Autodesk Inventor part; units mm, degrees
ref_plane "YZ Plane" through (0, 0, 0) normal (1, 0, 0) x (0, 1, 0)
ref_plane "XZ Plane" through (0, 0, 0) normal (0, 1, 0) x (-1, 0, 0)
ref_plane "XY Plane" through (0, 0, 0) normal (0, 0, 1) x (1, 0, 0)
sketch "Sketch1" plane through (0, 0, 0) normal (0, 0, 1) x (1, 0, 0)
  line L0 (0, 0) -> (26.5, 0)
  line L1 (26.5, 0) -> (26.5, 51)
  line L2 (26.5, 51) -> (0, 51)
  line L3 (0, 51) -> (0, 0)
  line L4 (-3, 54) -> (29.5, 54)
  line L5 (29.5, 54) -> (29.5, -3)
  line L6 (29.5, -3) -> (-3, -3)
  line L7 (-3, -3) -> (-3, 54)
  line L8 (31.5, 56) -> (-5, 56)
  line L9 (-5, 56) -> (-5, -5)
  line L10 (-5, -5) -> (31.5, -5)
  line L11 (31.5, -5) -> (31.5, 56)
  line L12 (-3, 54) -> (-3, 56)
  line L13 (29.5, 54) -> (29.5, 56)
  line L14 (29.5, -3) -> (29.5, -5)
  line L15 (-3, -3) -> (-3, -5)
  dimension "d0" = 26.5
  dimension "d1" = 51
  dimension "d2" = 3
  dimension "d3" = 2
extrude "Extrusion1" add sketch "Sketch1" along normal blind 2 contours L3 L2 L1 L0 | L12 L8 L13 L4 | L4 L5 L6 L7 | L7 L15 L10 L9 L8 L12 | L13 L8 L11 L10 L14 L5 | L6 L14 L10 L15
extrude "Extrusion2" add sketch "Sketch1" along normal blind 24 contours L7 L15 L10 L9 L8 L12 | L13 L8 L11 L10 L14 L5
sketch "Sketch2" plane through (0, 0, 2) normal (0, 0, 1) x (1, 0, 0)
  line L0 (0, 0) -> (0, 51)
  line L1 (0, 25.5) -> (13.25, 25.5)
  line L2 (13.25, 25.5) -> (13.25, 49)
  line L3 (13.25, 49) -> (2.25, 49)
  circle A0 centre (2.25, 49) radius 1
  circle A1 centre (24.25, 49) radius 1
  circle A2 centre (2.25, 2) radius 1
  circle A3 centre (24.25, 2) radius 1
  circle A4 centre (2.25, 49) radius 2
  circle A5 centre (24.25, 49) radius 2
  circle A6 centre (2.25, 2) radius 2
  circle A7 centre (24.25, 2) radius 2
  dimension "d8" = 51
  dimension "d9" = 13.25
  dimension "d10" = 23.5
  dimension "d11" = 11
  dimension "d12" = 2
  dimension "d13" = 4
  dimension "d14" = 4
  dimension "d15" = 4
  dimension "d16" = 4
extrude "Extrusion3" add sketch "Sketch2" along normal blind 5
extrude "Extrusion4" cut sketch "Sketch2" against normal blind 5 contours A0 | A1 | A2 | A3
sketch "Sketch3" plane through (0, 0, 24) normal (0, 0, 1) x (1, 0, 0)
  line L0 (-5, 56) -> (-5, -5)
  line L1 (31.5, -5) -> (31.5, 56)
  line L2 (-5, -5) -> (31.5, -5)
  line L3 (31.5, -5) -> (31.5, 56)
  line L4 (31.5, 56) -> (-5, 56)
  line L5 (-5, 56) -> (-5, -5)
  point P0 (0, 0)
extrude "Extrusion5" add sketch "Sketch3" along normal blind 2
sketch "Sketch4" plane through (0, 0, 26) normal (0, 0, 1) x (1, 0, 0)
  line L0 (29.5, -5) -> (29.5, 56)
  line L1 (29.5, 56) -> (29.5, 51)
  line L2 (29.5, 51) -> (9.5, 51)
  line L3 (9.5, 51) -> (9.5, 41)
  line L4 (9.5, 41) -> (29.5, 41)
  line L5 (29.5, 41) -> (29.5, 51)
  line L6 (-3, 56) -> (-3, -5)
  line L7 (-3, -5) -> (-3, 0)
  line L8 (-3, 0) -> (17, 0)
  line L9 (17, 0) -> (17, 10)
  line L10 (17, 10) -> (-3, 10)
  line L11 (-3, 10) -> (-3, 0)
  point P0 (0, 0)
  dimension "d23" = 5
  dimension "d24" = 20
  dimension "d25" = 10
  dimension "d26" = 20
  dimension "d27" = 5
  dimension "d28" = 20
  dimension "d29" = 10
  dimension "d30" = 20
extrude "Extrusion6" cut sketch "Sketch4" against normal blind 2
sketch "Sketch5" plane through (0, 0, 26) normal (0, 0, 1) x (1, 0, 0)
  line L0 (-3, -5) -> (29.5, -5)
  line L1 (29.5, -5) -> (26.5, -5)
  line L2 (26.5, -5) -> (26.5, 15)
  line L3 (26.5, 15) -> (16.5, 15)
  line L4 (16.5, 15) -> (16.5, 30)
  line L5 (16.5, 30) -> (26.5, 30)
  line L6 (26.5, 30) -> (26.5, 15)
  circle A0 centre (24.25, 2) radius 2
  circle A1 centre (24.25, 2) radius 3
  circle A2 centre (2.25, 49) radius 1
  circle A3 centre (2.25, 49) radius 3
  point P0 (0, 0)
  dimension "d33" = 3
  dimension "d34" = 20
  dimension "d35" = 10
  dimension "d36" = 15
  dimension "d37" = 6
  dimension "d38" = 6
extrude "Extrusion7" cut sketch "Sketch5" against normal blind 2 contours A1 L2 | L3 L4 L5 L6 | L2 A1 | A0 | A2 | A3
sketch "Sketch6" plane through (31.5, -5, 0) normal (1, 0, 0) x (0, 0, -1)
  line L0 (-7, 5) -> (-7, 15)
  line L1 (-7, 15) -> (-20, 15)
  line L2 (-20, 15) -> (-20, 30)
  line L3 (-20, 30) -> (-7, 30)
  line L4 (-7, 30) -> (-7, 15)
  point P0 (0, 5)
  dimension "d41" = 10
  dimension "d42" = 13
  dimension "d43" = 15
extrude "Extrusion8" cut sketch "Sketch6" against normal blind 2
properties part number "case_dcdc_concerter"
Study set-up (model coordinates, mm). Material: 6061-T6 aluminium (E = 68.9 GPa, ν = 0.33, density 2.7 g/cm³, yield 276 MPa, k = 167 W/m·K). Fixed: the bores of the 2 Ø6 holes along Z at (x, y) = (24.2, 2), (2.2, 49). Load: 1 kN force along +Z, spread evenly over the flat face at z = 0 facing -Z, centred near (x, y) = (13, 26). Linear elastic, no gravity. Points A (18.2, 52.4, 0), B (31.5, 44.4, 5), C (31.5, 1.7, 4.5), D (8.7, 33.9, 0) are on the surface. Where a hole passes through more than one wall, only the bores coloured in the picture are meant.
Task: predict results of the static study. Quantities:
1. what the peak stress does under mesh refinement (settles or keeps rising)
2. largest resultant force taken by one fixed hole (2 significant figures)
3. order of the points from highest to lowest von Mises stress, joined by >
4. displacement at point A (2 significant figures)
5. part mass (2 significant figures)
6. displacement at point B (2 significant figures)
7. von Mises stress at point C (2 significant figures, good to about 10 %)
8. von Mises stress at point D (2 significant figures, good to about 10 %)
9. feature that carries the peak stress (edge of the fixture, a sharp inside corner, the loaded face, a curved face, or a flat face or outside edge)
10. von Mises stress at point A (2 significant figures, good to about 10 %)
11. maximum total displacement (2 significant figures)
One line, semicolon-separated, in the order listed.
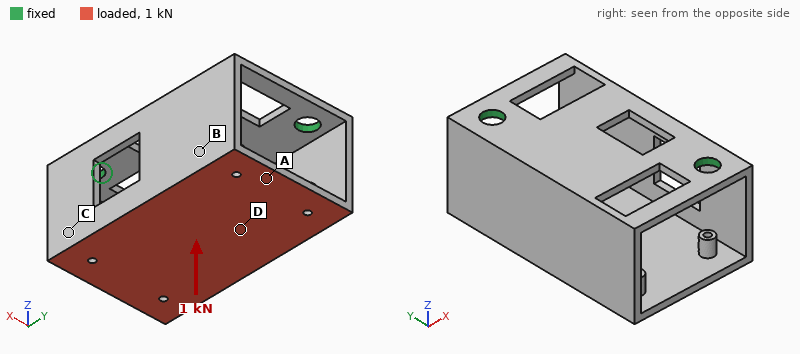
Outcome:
keeps rising; 520 N; C > A > D > B; 0.22 mm; 35 g; 0.17 mm; 80 MPa; 46 MPa; edge of the fixture; 62 MPa; 0.26 mm
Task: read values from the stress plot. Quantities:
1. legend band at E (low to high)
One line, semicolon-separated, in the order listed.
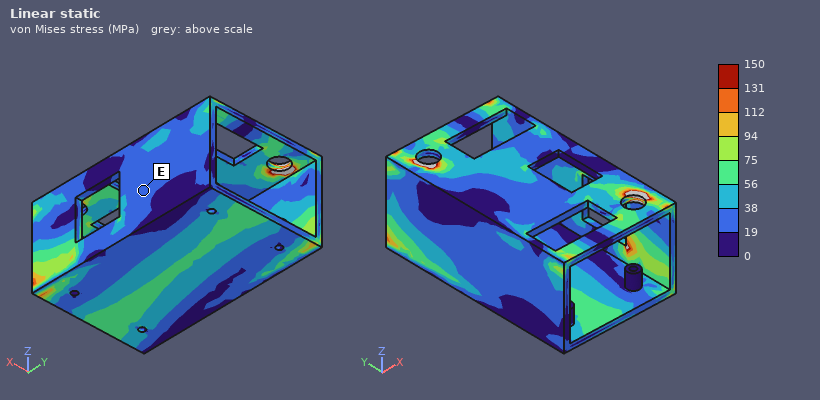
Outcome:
19 to 38 MPa
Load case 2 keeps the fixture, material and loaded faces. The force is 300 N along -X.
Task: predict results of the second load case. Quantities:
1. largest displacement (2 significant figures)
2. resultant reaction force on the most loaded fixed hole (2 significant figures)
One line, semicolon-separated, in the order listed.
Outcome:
0.49 mm; 180 N
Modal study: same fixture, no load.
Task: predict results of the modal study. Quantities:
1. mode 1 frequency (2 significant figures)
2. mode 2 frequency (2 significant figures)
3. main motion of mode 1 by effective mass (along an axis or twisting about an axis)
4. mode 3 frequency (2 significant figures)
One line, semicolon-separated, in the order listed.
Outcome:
900 Hz; 2100 Hz; along X; 2200 Hz
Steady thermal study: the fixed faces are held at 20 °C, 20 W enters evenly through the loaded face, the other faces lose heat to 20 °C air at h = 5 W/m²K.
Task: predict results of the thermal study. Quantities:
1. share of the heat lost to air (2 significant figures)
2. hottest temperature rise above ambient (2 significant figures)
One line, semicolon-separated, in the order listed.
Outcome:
5.5 %; 30 K
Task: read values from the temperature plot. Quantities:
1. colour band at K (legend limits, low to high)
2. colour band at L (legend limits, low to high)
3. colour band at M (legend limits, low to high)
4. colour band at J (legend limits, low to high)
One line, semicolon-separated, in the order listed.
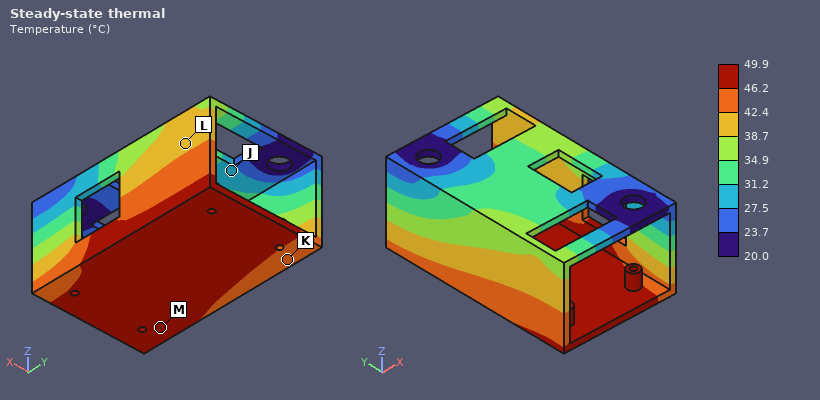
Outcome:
42.4 to 46.2 °C; 38.7 to 42.4 °C; 46.2 to 49.9 °C; 27.5 to 31.2 °C
